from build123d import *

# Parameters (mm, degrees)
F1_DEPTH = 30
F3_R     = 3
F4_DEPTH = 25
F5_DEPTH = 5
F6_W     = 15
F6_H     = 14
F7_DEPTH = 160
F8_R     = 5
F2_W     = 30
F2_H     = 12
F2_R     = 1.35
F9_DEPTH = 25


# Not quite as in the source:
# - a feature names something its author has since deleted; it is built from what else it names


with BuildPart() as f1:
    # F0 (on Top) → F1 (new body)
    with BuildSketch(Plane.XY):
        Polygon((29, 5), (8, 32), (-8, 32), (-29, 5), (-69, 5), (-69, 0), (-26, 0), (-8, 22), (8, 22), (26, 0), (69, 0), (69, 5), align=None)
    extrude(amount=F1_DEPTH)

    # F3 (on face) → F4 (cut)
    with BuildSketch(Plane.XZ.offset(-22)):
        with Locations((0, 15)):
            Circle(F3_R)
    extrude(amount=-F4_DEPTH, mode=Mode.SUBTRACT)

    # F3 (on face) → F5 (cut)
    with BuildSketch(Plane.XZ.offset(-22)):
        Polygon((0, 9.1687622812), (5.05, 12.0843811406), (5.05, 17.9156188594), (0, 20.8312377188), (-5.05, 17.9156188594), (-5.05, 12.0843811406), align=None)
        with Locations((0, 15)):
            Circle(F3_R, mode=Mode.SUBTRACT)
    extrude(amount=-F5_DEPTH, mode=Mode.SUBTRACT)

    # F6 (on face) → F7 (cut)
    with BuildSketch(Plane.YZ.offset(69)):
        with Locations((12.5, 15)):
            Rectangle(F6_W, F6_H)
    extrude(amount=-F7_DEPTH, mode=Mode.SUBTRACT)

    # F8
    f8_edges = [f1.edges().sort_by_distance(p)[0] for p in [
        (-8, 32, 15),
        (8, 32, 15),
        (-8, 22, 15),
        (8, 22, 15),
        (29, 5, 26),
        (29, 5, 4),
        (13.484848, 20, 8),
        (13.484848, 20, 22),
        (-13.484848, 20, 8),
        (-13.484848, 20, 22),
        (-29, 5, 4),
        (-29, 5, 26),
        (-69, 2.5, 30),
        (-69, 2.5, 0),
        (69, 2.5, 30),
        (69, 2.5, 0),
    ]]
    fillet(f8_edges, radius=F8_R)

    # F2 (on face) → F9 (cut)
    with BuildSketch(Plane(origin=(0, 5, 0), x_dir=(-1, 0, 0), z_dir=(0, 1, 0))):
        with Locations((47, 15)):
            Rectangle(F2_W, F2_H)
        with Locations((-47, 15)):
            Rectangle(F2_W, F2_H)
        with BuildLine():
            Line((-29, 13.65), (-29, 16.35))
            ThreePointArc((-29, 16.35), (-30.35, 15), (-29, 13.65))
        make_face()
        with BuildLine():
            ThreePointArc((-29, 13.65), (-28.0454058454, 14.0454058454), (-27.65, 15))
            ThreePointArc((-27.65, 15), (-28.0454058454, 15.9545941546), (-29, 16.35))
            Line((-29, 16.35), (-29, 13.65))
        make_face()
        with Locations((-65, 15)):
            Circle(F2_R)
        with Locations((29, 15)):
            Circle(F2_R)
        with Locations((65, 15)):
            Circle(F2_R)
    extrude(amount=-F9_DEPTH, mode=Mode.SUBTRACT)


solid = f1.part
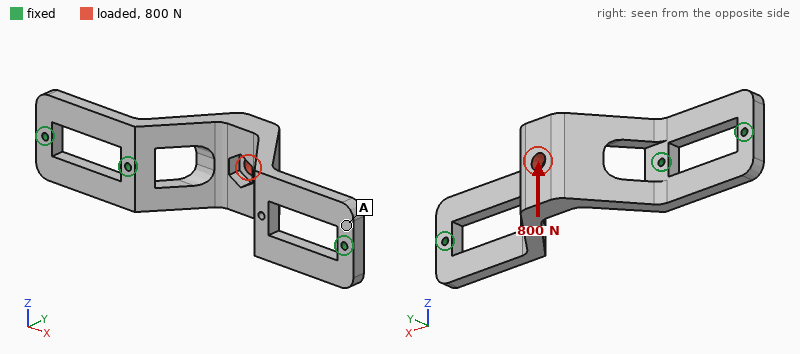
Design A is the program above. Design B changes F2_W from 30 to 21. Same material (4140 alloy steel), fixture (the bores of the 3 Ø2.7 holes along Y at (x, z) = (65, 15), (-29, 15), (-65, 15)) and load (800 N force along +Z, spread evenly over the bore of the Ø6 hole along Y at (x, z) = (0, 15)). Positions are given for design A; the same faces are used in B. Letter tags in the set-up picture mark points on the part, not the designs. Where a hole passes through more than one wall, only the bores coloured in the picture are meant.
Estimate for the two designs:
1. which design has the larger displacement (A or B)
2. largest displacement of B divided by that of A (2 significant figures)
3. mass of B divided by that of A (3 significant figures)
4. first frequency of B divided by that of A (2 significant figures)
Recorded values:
A
0.86
1.05
1.1
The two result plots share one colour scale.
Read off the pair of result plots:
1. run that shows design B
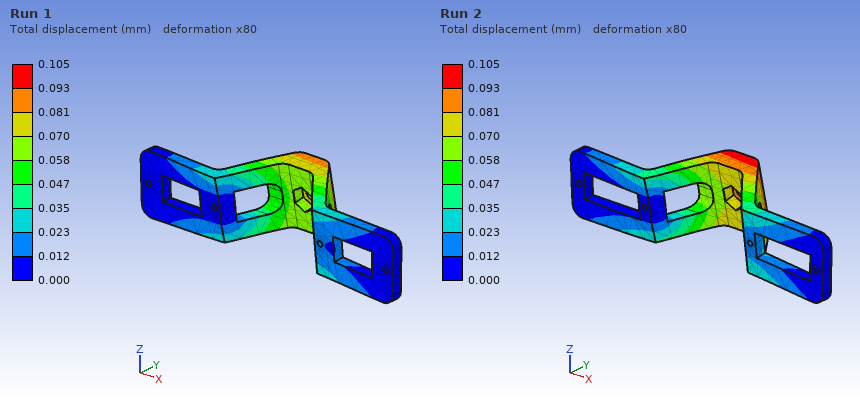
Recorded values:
Run 1
